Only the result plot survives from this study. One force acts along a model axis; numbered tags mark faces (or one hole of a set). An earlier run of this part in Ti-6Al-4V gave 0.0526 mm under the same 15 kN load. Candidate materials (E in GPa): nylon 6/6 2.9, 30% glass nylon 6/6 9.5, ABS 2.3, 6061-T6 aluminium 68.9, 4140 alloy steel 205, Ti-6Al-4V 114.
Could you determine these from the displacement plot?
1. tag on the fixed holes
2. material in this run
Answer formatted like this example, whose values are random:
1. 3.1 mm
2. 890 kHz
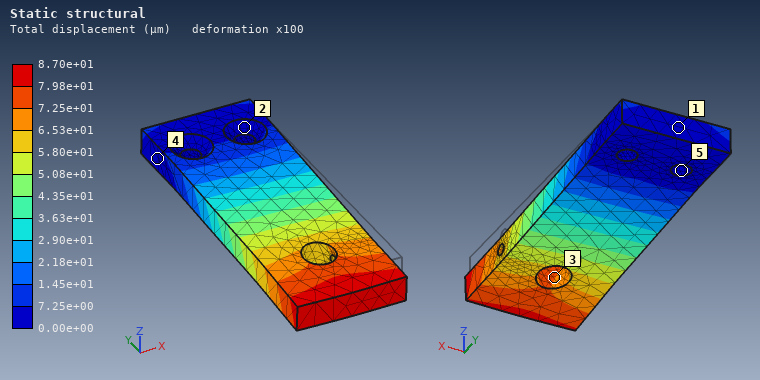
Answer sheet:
1. 5
2. 6061-T6 aluminium
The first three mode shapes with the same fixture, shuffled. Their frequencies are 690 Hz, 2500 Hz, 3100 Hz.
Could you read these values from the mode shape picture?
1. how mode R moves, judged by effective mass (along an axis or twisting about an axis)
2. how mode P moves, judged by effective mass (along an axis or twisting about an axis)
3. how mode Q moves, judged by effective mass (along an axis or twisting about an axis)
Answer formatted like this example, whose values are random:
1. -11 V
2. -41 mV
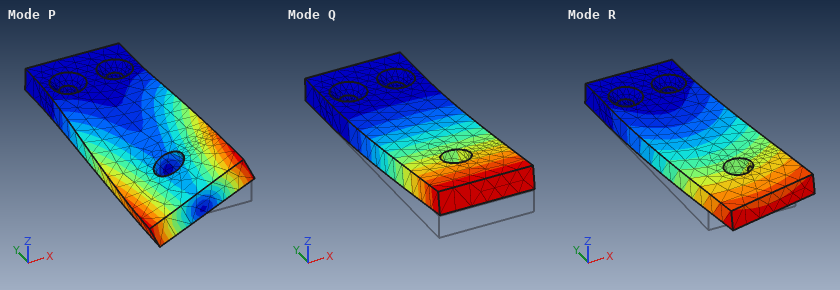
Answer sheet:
1. along X
2. twisting about Y
3. along Z
